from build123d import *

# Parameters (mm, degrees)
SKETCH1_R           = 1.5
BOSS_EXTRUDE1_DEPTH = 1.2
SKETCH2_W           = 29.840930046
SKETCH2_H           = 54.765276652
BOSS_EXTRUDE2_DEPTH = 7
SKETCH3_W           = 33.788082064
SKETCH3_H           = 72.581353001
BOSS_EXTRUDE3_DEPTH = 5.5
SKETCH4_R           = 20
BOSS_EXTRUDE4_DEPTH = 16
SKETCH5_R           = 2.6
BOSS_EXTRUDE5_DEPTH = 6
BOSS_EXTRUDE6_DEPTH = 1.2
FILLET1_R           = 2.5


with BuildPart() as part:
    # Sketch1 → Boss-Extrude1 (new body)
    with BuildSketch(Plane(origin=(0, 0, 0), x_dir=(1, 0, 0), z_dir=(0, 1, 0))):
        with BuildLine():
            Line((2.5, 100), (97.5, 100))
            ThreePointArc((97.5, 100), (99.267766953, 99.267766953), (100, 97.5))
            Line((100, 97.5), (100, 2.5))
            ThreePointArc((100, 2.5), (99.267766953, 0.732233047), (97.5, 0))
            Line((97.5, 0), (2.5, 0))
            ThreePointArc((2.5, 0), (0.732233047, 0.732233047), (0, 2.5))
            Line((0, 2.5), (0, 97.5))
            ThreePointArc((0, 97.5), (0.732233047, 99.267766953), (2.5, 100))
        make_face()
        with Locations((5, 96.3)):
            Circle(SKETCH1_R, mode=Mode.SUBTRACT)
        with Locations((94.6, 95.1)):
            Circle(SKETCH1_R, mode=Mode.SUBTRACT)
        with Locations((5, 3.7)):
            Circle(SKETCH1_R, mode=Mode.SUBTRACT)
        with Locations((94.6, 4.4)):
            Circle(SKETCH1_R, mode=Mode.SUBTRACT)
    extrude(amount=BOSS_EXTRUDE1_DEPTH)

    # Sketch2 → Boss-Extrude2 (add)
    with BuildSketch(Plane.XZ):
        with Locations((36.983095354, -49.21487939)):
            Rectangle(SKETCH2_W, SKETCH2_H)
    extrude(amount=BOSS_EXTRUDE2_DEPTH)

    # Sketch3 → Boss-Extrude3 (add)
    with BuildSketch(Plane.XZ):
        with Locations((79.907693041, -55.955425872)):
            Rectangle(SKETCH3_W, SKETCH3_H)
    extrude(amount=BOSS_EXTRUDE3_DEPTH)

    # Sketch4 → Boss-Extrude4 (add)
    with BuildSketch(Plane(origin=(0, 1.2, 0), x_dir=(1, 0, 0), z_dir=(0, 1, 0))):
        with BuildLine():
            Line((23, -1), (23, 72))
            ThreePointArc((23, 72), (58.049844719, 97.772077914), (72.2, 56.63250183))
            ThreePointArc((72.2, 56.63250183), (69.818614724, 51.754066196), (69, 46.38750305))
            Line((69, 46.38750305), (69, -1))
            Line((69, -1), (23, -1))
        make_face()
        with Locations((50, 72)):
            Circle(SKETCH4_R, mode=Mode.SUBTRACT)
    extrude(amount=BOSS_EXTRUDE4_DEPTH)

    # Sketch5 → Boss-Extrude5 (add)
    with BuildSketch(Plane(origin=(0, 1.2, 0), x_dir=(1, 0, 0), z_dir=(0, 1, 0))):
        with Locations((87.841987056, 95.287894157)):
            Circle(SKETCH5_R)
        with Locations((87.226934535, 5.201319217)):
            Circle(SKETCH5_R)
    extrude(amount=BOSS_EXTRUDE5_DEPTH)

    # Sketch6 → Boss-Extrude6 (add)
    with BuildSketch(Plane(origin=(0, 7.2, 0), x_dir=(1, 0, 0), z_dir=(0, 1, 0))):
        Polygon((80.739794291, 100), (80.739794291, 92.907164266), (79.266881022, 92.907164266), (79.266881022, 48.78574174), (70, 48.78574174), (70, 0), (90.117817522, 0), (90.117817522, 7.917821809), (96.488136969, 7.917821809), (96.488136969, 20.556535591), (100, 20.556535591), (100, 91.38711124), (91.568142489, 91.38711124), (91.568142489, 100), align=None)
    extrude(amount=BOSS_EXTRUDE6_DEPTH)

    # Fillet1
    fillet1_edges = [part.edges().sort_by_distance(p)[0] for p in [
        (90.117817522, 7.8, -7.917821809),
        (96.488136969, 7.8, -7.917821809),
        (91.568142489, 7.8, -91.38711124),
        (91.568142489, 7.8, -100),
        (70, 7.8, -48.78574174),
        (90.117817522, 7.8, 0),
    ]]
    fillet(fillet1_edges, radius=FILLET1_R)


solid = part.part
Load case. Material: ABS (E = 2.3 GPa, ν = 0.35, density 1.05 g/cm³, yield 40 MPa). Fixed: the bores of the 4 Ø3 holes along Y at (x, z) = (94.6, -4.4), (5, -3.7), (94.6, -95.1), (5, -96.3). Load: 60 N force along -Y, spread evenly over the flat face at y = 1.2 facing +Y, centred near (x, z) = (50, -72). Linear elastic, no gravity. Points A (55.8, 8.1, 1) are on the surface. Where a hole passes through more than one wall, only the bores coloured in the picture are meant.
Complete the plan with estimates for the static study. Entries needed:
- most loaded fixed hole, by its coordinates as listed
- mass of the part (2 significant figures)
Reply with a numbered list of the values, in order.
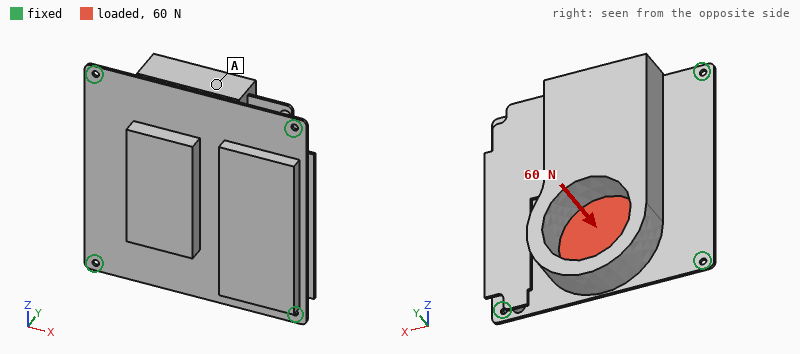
1. (94.6, -95.1)
2. 98 g
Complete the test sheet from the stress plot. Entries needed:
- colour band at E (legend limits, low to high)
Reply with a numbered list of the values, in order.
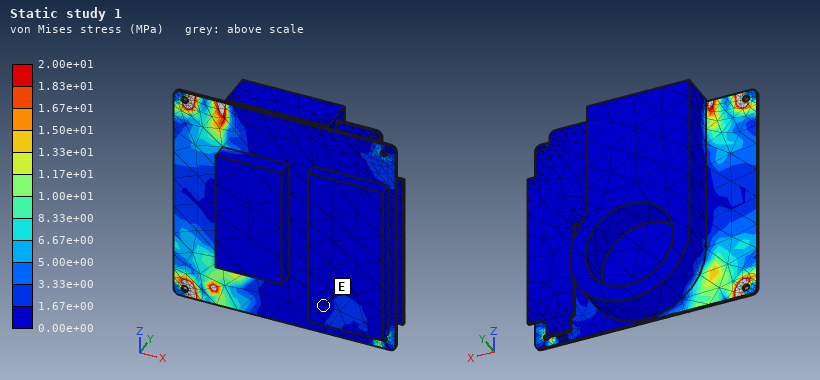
1. 0.00e+00 to 1.67e+00 MPa
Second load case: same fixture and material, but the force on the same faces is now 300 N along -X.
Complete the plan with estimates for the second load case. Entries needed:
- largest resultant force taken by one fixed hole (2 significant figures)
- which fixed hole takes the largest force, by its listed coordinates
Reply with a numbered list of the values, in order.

1. 120 N
2. (94.6, -95.1)
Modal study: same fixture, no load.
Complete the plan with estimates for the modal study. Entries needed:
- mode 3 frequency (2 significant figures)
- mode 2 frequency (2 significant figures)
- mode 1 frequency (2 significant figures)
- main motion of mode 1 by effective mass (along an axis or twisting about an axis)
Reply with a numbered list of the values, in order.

1. 230 Hz
2. 200 Hz
3. 130 Hz
4. along Y
